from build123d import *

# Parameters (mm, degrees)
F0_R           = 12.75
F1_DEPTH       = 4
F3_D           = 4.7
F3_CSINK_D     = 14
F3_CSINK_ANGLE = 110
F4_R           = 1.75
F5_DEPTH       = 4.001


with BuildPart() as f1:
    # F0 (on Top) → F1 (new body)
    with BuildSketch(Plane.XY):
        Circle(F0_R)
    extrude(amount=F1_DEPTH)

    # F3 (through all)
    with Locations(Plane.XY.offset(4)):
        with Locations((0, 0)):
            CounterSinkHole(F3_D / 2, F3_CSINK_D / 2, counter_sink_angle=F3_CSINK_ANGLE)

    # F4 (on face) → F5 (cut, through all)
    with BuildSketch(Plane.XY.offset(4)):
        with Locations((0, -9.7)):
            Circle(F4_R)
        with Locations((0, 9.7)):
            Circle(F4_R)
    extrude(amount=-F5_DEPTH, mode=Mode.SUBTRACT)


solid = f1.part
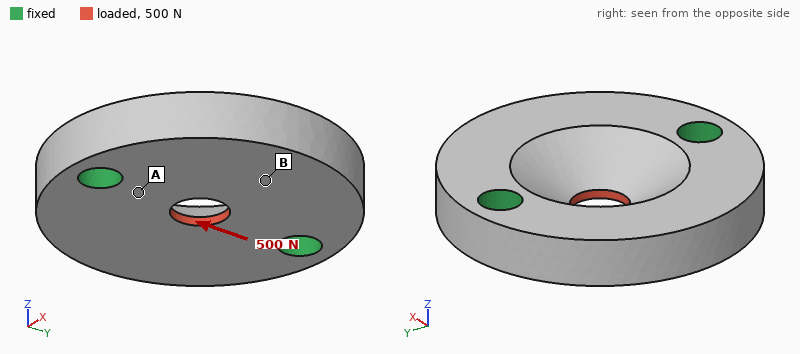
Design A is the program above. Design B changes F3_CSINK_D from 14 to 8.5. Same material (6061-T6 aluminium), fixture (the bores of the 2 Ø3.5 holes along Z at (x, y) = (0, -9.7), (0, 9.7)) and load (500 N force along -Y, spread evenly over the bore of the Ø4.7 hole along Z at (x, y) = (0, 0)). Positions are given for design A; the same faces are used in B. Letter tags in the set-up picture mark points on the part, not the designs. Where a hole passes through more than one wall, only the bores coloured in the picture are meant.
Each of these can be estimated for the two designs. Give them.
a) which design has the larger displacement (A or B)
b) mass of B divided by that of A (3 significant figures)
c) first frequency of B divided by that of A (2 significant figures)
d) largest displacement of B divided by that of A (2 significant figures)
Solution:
A
1.09
1.0
0.38
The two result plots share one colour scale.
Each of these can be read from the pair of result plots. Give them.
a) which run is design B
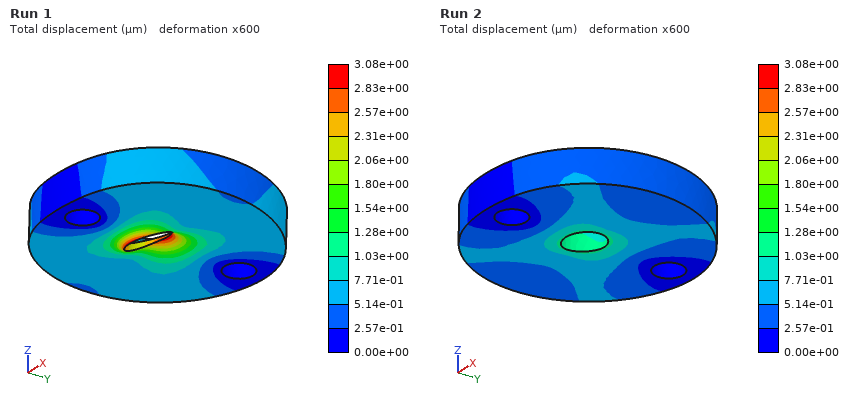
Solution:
Run 2
